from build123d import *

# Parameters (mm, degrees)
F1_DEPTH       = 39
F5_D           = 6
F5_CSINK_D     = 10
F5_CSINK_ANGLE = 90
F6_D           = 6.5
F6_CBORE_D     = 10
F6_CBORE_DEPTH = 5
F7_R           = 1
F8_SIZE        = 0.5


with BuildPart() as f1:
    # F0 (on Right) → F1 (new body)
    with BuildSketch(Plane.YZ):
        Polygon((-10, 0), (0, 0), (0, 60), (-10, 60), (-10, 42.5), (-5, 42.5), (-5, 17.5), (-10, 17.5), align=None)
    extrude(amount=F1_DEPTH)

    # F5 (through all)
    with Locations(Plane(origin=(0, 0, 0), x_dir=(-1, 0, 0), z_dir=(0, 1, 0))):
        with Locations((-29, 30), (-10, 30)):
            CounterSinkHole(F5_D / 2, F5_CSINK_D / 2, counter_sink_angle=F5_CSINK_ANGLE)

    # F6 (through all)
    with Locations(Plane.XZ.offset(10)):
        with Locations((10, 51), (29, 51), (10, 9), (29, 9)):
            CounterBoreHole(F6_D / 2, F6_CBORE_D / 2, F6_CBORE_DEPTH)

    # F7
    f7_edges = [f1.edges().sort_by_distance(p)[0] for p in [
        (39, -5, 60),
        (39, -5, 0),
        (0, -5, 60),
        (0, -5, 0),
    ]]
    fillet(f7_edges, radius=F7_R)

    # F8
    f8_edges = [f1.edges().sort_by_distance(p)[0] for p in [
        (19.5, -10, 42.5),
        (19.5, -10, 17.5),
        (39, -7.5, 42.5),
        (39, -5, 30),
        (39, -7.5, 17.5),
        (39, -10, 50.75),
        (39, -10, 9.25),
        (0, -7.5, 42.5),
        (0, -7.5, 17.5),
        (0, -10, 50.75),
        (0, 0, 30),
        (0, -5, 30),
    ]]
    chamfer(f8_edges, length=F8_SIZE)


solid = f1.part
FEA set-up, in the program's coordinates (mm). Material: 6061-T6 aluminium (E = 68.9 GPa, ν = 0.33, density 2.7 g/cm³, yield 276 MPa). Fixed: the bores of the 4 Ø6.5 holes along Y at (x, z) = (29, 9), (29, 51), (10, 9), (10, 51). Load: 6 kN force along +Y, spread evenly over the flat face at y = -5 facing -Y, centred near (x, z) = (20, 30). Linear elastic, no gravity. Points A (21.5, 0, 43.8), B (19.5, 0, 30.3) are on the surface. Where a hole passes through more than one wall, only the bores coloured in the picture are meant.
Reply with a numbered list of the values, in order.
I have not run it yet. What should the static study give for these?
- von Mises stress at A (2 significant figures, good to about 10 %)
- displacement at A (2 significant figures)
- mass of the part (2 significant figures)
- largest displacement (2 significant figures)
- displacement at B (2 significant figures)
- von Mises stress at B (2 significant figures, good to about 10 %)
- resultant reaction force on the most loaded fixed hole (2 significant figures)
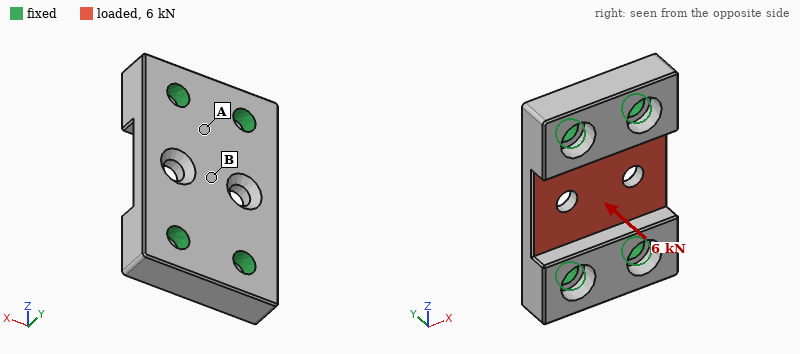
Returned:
1. 37 MPa
2. 15 µm
3. 43 g
4. 49 µm
5. 45 µm
6. 81 MPa
7. 1.5 kN
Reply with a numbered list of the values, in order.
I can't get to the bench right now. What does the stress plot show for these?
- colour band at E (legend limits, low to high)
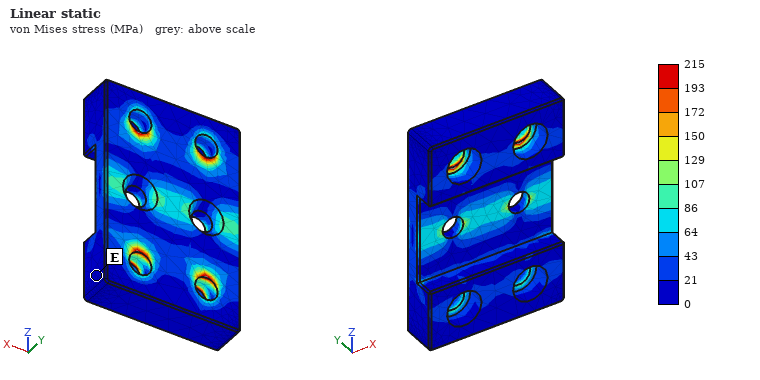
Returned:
1. 0 to 21 MPa
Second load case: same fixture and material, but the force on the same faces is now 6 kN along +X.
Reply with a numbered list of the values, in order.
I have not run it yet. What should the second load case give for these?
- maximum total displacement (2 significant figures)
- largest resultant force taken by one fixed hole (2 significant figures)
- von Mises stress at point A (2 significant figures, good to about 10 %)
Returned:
1. 17 µm
2. 1.7 kN
3. 25 MPa
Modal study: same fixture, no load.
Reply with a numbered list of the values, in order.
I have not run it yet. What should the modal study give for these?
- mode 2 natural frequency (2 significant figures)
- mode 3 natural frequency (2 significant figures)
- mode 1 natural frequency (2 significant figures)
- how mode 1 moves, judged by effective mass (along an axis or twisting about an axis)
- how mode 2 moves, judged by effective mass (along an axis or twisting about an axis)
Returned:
1. 20 kHz
2. 30 kHz
3. 17 kHz
4. along Y
5. twisting about Z
